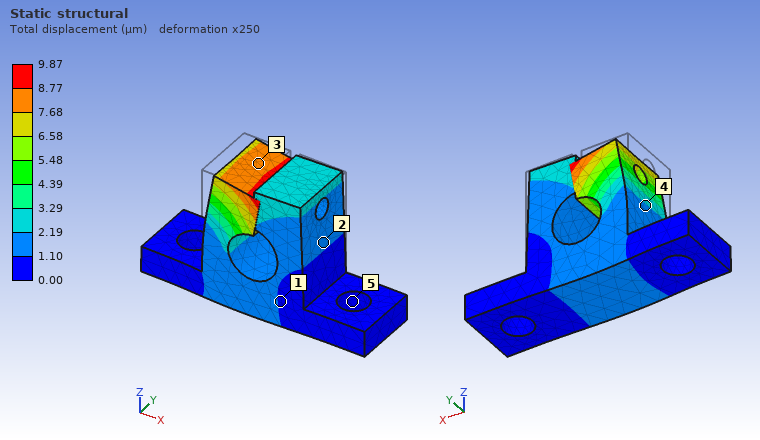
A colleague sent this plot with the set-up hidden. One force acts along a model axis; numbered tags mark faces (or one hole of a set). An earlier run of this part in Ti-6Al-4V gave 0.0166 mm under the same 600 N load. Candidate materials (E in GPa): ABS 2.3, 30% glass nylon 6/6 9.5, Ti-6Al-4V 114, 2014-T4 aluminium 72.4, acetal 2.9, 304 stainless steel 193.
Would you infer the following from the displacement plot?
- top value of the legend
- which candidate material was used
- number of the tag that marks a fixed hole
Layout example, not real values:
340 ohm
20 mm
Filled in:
9.87 µm
304 stainless steel
5
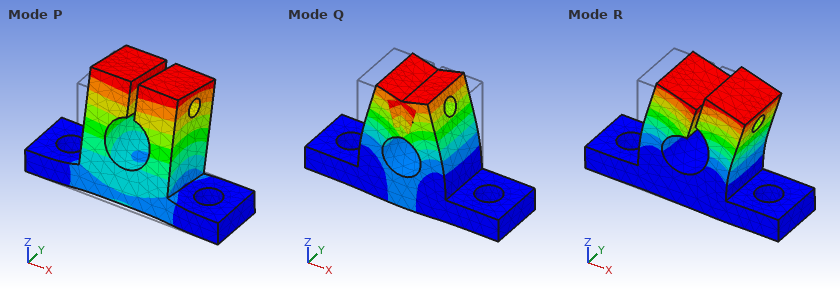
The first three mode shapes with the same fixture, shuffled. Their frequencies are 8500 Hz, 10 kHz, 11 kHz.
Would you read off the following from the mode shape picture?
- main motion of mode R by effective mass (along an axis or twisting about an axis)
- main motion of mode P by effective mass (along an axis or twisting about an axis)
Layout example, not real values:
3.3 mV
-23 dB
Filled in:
along X
along Y
